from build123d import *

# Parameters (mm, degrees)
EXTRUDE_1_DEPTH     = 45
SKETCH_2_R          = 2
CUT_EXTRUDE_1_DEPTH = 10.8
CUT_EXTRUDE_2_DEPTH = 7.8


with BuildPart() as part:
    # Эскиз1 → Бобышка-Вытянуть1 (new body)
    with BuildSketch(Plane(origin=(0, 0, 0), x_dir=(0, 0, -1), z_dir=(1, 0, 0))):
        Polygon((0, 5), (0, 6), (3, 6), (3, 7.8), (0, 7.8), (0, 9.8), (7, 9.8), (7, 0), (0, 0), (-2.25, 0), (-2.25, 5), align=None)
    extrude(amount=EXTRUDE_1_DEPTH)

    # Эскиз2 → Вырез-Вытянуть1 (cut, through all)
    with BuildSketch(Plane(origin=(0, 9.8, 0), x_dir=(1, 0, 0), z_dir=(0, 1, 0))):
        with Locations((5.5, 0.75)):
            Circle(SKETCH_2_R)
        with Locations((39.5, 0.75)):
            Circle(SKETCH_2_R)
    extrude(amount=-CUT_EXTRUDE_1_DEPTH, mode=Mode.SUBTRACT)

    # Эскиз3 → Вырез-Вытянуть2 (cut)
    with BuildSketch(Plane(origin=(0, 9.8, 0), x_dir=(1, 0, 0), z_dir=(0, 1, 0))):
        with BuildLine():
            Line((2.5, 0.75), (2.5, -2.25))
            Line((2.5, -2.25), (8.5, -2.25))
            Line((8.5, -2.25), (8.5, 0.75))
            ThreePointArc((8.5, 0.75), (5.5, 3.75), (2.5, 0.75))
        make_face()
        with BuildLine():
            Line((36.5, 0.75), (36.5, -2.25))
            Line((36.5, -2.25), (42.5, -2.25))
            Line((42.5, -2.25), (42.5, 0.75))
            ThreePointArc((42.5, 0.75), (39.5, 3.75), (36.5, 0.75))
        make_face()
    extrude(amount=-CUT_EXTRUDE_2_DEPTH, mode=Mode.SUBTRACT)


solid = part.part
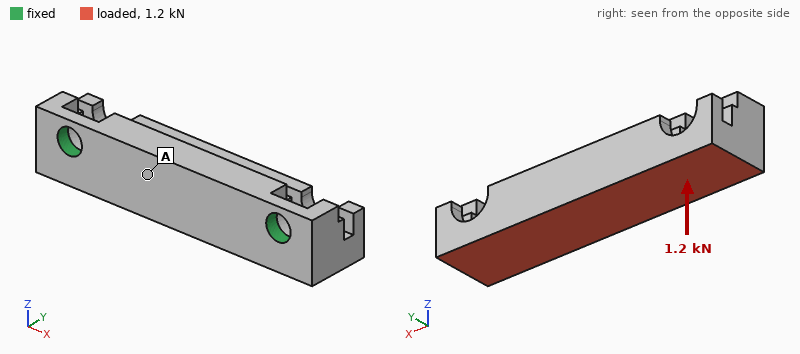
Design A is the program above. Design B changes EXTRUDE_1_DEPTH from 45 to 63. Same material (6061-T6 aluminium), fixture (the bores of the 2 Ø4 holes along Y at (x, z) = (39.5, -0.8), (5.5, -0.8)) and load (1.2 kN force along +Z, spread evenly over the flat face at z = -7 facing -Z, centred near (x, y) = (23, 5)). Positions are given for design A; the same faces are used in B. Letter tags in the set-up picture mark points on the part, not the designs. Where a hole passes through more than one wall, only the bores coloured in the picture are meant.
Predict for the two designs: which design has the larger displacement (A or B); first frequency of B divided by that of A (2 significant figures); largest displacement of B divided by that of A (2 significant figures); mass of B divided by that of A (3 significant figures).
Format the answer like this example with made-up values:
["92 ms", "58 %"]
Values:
["B", "0.52", "2.2", "1.45"]
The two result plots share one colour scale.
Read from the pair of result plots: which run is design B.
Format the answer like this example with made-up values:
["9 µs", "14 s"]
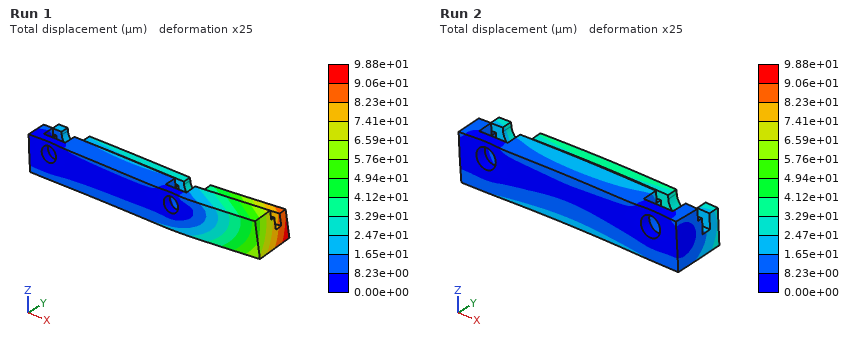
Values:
["Run 1"]
